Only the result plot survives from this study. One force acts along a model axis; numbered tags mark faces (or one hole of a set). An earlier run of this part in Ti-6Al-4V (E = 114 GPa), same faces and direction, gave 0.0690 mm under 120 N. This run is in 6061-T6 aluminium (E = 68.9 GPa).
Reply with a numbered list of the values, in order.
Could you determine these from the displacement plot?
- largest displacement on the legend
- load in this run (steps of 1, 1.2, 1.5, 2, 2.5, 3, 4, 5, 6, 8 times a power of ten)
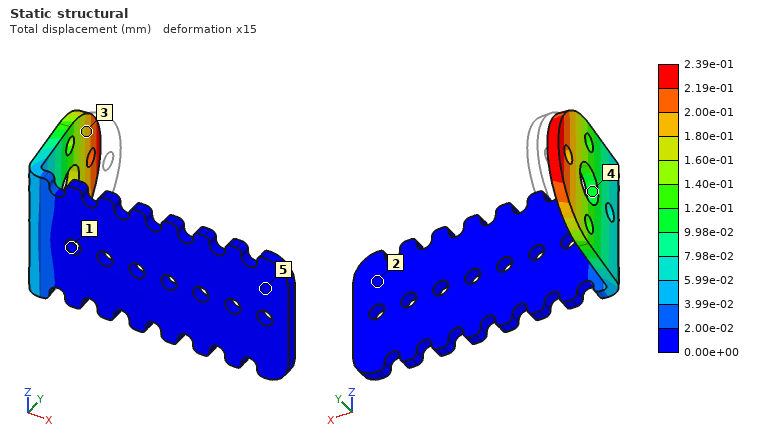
1. 2.39e-01 mm
2. 250 N
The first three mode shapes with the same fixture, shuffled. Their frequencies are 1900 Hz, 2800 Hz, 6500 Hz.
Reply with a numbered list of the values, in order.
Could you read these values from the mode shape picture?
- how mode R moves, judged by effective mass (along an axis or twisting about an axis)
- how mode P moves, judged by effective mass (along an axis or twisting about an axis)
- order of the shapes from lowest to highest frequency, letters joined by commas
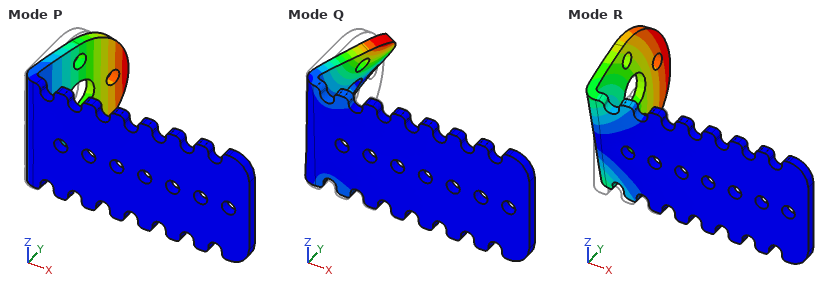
1. along Z
2. along X
3. P, R, Q
